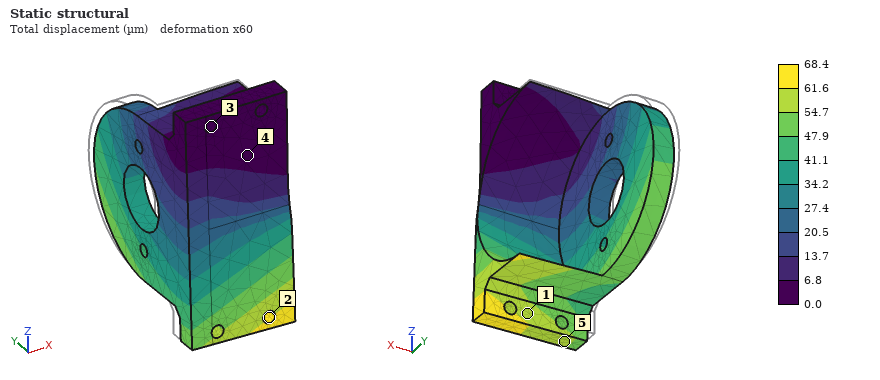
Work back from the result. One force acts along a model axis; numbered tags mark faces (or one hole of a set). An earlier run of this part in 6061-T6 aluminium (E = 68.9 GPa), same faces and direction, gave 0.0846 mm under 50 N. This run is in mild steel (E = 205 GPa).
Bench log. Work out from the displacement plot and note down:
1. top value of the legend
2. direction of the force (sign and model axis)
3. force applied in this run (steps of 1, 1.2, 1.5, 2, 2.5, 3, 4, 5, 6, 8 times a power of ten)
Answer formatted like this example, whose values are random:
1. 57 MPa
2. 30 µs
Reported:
1. 68.4 µm
2. -Y
3. 120 N
